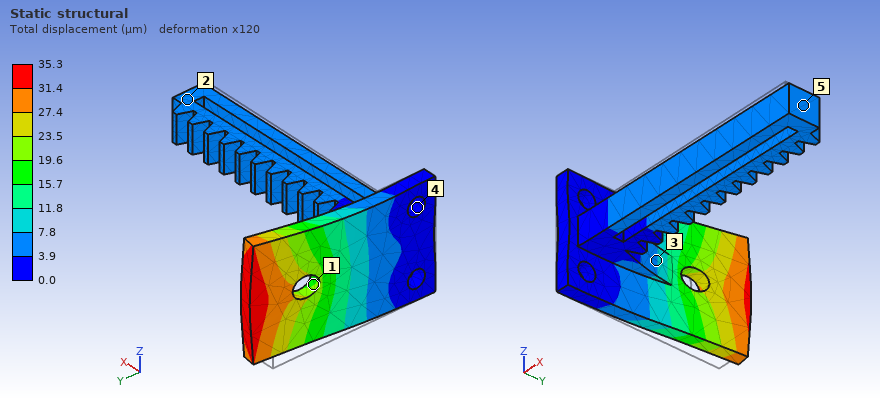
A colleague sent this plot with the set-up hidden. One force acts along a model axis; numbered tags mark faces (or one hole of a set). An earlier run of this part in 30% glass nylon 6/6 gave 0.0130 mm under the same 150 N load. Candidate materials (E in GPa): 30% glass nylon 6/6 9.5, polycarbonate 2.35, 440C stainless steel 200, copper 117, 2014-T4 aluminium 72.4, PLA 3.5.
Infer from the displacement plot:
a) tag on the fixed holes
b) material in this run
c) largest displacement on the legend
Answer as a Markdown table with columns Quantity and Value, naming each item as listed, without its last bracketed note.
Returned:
| Quantity | Value |
|---|---|
| tag on the fixed holes | 4 |
| material in this run | PLA |
| largest displacement on the legend | 35.3 µm |
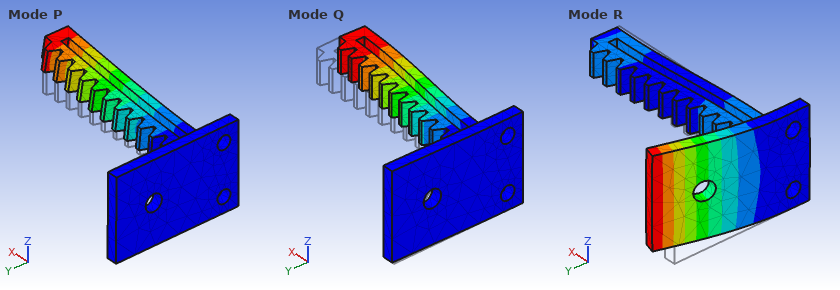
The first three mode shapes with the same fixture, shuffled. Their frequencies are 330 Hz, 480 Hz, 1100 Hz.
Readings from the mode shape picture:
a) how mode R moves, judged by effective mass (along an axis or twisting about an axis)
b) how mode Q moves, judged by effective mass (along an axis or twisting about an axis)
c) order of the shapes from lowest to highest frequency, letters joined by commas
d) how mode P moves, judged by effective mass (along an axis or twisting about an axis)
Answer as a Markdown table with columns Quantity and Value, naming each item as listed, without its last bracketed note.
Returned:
| Quantity | Value |
|---|---|
| how mode R moves, judged by effective mass | along X |
| how mode Q moves, judged by effective mass | along Y |
| order of the shapes from lowest to highest frequency, letters joined by commas | Q, P, R |
| how mode P moves, judged by effective mass | along Z |
